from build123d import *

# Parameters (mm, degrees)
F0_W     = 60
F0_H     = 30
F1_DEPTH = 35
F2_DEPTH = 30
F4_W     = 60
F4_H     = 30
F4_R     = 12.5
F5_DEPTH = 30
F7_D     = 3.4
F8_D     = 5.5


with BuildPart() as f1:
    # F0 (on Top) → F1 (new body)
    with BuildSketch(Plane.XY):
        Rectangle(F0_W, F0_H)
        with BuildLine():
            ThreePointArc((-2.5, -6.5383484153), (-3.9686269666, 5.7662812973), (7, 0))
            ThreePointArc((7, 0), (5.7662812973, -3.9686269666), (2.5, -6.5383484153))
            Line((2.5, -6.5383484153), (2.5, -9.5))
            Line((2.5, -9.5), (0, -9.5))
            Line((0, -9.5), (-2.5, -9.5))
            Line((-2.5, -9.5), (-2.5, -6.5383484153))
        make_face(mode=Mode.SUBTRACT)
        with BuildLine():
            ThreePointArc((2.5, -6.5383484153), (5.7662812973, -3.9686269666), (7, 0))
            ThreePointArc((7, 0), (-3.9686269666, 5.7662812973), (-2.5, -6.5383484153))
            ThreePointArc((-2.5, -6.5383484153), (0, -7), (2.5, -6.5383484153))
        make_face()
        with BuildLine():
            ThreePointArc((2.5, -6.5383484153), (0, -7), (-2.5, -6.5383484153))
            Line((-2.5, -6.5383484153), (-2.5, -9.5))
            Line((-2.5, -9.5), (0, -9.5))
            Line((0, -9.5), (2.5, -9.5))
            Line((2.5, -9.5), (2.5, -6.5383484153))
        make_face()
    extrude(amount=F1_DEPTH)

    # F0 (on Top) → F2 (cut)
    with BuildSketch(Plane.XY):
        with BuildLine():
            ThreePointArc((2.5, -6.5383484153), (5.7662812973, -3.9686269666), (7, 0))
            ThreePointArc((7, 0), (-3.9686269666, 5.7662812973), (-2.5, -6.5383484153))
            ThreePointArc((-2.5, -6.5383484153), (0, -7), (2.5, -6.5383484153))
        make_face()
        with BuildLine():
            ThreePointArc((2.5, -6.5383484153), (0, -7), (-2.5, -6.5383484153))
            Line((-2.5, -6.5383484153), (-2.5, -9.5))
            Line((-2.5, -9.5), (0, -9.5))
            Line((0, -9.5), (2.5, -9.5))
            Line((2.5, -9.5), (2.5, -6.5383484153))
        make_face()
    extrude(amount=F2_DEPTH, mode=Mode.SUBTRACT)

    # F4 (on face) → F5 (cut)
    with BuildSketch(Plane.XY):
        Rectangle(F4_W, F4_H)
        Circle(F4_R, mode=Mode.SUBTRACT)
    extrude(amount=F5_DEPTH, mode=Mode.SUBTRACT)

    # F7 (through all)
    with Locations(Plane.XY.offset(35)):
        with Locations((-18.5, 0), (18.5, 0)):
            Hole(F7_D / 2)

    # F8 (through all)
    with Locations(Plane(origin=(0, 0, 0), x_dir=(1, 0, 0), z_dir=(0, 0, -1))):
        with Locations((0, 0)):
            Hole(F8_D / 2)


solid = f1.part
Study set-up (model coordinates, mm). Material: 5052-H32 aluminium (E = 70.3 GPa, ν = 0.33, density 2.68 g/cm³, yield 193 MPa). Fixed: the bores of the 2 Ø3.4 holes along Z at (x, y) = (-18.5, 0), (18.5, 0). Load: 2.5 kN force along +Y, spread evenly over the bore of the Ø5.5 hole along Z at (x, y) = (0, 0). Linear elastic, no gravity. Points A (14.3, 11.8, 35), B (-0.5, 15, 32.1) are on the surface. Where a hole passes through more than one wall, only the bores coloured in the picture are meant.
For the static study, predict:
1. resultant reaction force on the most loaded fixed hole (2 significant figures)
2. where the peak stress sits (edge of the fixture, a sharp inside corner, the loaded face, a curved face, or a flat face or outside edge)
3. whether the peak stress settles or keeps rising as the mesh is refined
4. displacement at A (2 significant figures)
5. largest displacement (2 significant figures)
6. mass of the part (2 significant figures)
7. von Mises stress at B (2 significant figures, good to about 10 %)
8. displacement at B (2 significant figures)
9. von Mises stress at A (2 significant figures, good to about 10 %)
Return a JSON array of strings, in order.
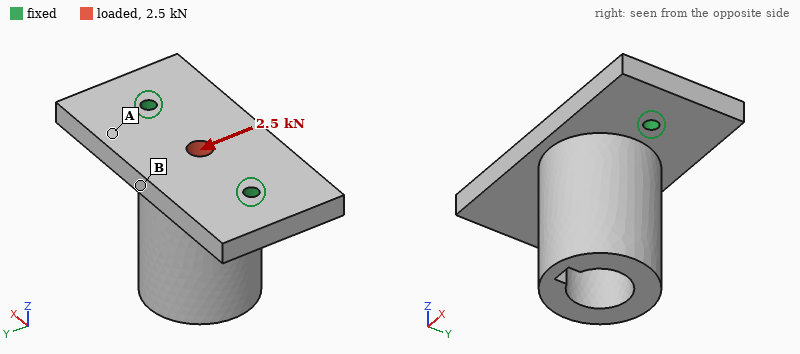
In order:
["1.3 kN", "edge of the fixture", "keeps rising", "3.8 µm", "9.9 µm", "50 g", "26 MPa", "7.1 µm", "9.5 MPa"]
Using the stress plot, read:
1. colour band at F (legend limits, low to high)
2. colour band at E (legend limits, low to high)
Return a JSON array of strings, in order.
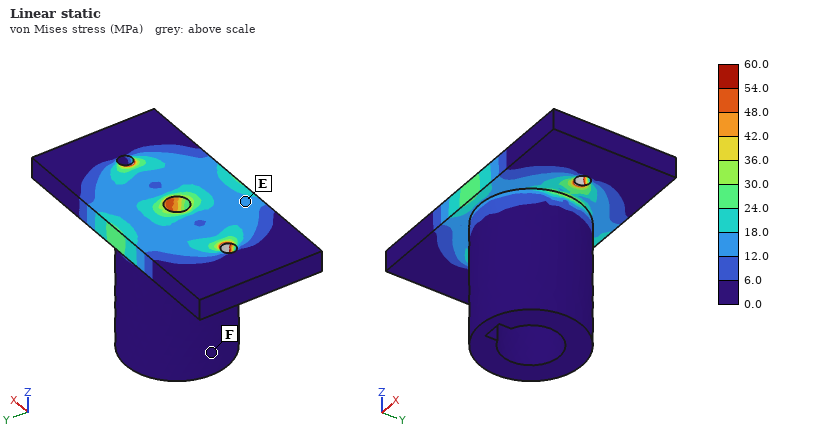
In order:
["0.0 to 6.0 MPa", "12.0 to 18.0 MPa"]
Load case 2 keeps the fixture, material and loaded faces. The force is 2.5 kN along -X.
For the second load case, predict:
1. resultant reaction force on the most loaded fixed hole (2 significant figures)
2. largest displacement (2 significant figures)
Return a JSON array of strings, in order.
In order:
["1.3 kN", "5.0 µm"]
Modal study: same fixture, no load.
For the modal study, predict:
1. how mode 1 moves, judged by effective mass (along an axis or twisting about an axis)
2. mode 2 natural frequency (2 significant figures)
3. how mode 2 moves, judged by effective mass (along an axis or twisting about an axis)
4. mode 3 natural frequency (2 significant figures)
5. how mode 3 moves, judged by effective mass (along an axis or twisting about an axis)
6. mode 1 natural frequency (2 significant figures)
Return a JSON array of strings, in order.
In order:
["along Y", "8500 Hz", "along X", "11 kHz", "along Z", "3300 Hz"]
